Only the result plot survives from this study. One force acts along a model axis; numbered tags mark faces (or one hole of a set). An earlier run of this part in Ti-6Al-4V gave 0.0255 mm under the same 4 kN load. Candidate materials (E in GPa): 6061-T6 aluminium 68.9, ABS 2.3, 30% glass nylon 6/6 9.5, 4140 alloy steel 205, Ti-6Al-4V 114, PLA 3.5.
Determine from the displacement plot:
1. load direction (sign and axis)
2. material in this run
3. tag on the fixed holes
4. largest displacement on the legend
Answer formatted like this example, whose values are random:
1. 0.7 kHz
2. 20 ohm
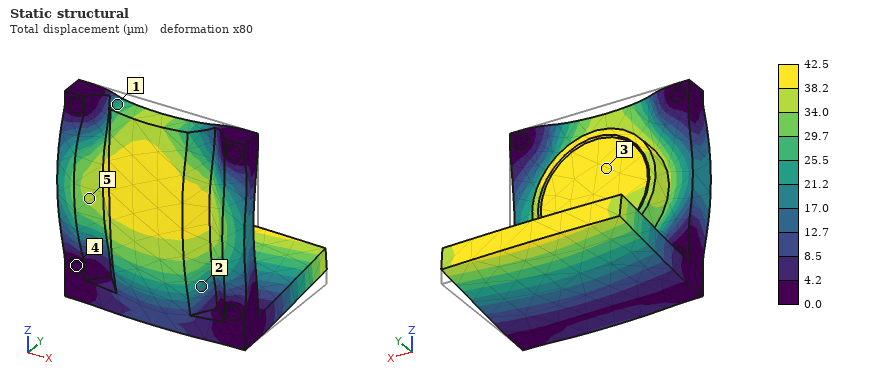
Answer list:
1. -Y
2. 6061-T6 aluminium
3. 4
4. 42.5 µm
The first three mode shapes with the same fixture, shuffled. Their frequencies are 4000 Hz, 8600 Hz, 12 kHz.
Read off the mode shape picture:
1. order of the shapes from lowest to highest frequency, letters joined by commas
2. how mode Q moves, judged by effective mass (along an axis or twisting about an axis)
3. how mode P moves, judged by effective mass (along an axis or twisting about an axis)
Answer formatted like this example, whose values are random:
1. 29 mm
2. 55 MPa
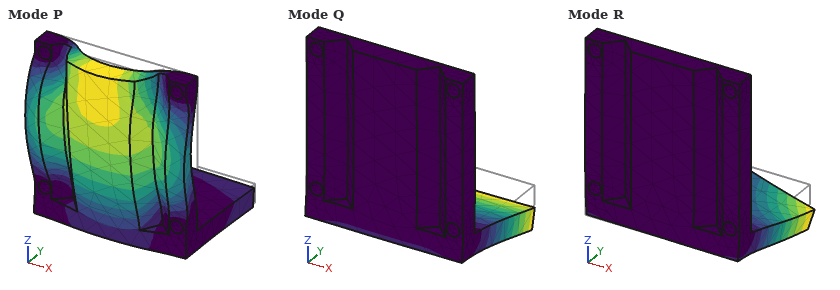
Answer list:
1. Q, R, P
2. along Z
3. along Y
